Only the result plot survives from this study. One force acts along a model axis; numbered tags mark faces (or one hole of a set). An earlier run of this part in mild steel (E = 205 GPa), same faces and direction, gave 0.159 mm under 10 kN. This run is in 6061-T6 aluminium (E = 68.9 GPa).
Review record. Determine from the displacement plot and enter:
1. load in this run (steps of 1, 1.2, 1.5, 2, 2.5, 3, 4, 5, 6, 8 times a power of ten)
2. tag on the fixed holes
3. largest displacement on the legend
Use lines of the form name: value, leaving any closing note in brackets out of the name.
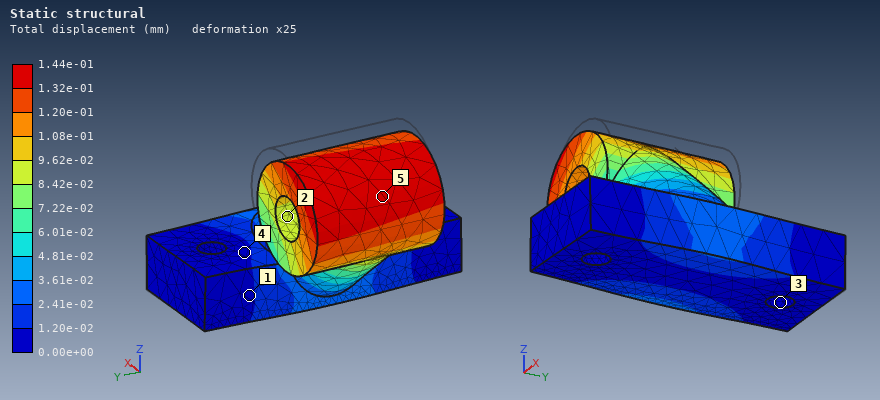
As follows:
load in this run: 3 kN
tag on the fixed holes: 3
largest displacement on the legend: 1.44e-01 mm
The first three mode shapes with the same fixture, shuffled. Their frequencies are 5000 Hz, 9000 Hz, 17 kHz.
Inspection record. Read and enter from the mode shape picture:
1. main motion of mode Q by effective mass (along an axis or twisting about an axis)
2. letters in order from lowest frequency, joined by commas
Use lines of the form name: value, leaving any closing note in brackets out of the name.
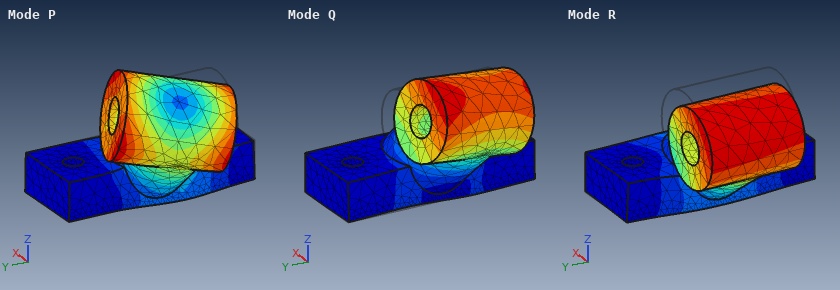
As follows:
main motion of mode Q by effective mass: along Y
letters in order from lowest frequency, joined by commas: R, Q, P
